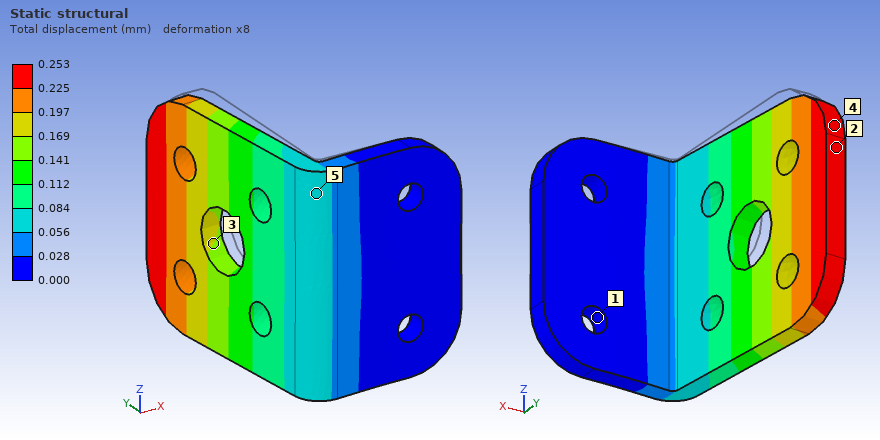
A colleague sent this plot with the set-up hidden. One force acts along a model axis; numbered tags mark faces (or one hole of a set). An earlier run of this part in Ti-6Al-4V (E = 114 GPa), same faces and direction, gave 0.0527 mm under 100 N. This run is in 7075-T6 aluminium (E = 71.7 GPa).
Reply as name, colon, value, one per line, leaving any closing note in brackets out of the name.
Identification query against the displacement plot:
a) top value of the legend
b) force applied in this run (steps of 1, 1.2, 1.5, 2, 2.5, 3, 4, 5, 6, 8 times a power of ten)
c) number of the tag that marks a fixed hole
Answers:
top value of the legend: 0.253 mm
force applied in this run: 300 N
number of the tag that marks a fixed hole: 1
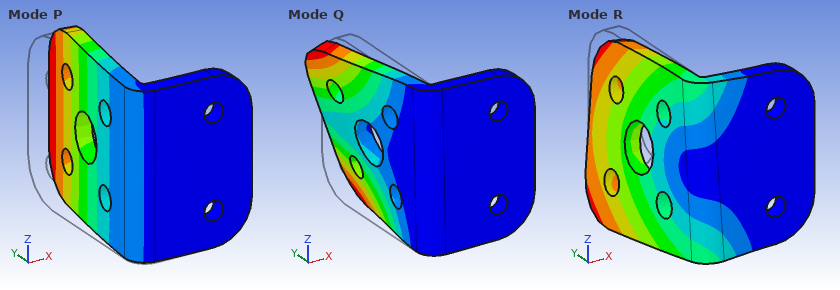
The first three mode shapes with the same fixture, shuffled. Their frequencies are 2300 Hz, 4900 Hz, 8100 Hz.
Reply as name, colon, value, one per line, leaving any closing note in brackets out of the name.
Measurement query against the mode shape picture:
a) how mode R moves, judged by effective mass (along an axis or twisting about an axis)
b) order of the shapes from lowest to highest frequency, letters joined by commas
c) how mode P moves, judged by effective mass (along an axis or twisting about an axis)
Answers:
how mode R moves, judged by effective mass: along Z
order of the shapes from lowest to highest frequency, letters joined by commas: P, R, Q
how mode P moves, judged by effective mass: along X
